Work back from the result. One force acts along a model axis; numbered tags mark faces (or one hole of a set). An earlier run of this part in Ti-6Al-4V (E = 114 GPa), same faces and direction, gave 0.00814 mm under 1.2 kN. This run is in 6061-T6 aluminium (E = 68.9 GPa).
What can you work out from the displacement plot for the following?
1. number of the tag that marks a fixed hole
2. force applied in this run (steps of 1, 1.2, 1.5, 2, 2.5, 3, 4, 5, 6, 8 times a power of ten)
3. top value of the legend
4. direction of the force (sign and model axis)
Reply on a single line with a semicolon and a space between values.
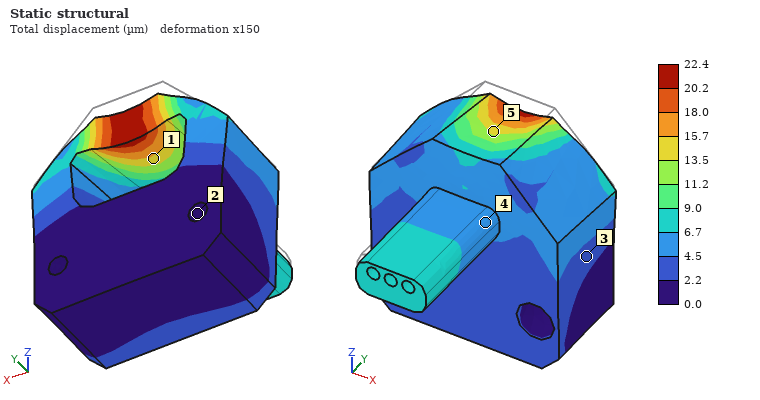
2; 2 kN; 22.4 µm; -Z
